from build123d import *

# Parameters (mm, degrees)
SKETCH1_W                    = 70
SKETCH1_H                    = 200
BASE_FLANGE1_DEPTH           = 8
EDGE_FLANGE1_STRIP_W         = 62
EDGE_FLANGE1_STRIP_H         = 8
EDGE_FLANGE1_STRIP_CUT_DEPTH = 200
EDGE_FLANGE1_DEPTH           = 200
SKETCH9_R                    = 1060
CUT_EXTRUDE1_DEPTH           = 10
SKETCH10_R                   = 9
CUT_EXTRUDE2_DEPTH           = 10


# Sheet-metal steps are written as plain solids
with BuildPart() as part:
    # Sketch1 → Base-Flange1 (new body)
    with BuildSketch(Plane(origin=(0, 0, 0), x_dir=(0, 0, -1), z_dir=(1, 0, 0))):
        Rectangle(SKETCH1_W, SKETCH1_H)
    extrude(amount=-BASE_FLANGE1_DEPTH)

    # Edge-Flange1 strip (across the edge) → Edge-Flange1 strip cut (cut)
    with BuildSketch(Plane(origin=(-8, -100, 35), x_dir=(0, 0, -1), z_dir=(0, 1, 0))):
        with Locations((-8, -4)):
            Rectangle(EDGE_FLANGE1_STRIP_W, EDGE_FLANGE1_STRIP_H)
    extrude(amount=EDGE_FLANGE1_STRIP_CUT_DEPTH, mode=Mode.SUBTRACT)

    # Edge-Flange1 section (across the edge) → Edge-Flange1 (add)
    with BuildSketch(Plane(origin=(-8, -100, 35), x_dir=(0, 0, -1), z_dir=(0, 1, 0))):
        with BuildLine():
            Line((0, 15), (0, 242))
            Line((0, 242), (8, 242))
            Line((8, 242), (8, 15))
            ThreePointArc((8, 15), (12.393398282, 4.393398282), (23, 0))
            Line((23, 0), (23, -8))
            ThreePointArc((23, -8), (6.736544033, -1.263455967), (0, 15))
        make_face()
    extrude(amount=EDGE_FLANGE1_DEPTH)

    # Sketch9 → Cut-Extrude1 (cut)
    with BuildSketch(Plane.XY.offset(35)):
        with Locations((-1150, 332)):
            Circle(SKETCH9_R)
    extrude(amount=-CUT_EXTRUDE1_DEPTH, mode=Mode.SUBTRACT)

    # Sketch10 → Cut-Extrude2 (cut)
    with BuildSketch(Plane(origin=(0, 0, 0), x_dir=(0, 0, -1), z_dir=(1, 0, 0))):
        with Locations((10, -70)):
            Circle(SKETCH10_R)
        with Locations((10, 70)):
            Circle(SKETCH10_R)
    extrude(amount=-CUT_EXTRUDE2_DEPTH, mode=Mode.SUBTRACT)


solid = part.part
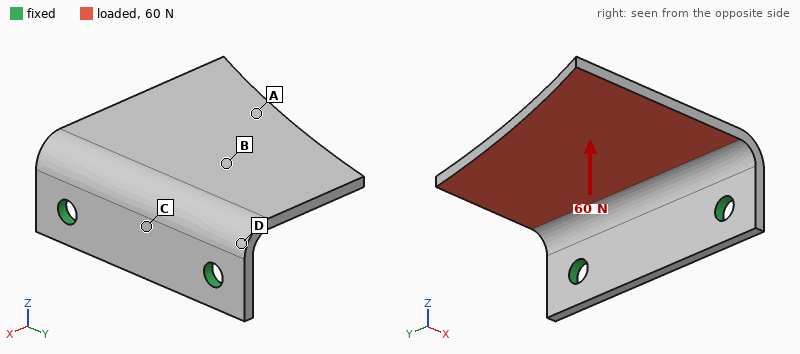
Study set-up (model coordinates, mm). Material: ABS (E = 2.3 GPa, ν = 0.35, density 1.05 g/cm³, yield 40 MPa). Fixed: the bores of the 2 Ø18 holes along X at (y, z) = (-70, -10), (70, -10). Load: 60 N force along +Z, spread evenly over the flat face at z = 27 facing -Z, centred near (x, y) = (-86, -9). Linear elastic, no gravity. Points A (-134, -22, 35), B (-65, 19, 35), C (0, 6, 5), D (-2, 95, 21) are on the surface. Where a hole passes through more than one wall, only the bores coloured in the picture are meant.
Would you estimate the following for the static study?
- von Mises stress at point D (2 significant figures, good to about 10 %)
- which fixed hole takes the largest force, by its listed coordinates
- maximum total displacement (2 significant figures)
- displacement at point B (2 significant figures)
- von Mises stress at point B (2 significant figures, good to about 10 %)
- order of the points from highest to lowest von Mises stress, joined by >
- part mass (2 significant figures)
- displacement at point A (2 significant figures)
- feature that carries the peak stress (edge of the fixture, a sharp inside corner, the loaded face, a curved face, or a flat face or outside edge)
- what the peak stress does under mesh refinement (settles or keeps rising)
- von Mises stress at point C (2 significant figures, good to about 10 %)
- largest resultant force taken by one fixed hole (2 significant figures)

1.7 MPa
(-70, -10)
3.2 mm
0.82 mm
0.71 MPa
D > C > B > A
330 g
2.1 mm
edge of the fixture
keeps rising
1.2 MPa
35 N
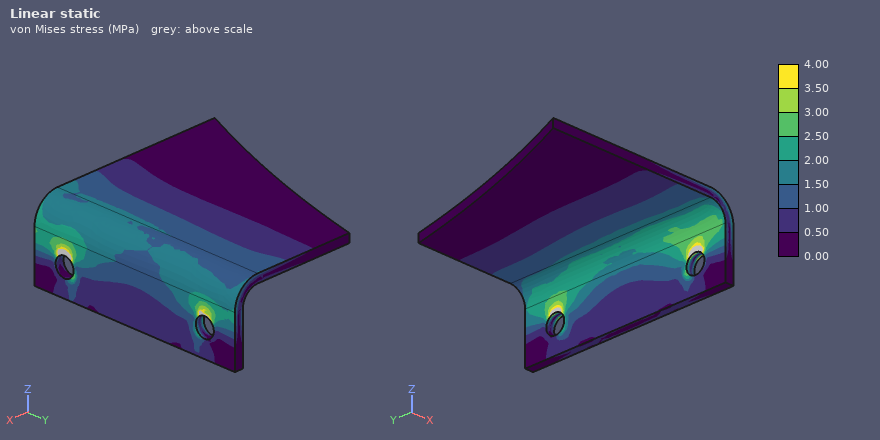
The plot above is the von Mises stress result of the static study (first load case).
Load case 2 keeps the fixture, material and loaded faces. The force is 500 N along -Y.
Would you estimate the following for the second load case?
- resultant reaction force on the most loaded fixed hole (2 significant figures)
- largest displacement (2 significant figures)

390 N
2.2 mm
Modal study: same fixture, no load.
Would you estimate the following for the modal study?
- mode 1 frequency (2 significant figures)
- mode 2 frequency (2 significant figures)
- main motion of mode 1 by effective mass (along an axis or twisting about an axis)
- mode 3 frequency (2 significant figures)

67 Hz
160 Hz
along Z
280 Hz
